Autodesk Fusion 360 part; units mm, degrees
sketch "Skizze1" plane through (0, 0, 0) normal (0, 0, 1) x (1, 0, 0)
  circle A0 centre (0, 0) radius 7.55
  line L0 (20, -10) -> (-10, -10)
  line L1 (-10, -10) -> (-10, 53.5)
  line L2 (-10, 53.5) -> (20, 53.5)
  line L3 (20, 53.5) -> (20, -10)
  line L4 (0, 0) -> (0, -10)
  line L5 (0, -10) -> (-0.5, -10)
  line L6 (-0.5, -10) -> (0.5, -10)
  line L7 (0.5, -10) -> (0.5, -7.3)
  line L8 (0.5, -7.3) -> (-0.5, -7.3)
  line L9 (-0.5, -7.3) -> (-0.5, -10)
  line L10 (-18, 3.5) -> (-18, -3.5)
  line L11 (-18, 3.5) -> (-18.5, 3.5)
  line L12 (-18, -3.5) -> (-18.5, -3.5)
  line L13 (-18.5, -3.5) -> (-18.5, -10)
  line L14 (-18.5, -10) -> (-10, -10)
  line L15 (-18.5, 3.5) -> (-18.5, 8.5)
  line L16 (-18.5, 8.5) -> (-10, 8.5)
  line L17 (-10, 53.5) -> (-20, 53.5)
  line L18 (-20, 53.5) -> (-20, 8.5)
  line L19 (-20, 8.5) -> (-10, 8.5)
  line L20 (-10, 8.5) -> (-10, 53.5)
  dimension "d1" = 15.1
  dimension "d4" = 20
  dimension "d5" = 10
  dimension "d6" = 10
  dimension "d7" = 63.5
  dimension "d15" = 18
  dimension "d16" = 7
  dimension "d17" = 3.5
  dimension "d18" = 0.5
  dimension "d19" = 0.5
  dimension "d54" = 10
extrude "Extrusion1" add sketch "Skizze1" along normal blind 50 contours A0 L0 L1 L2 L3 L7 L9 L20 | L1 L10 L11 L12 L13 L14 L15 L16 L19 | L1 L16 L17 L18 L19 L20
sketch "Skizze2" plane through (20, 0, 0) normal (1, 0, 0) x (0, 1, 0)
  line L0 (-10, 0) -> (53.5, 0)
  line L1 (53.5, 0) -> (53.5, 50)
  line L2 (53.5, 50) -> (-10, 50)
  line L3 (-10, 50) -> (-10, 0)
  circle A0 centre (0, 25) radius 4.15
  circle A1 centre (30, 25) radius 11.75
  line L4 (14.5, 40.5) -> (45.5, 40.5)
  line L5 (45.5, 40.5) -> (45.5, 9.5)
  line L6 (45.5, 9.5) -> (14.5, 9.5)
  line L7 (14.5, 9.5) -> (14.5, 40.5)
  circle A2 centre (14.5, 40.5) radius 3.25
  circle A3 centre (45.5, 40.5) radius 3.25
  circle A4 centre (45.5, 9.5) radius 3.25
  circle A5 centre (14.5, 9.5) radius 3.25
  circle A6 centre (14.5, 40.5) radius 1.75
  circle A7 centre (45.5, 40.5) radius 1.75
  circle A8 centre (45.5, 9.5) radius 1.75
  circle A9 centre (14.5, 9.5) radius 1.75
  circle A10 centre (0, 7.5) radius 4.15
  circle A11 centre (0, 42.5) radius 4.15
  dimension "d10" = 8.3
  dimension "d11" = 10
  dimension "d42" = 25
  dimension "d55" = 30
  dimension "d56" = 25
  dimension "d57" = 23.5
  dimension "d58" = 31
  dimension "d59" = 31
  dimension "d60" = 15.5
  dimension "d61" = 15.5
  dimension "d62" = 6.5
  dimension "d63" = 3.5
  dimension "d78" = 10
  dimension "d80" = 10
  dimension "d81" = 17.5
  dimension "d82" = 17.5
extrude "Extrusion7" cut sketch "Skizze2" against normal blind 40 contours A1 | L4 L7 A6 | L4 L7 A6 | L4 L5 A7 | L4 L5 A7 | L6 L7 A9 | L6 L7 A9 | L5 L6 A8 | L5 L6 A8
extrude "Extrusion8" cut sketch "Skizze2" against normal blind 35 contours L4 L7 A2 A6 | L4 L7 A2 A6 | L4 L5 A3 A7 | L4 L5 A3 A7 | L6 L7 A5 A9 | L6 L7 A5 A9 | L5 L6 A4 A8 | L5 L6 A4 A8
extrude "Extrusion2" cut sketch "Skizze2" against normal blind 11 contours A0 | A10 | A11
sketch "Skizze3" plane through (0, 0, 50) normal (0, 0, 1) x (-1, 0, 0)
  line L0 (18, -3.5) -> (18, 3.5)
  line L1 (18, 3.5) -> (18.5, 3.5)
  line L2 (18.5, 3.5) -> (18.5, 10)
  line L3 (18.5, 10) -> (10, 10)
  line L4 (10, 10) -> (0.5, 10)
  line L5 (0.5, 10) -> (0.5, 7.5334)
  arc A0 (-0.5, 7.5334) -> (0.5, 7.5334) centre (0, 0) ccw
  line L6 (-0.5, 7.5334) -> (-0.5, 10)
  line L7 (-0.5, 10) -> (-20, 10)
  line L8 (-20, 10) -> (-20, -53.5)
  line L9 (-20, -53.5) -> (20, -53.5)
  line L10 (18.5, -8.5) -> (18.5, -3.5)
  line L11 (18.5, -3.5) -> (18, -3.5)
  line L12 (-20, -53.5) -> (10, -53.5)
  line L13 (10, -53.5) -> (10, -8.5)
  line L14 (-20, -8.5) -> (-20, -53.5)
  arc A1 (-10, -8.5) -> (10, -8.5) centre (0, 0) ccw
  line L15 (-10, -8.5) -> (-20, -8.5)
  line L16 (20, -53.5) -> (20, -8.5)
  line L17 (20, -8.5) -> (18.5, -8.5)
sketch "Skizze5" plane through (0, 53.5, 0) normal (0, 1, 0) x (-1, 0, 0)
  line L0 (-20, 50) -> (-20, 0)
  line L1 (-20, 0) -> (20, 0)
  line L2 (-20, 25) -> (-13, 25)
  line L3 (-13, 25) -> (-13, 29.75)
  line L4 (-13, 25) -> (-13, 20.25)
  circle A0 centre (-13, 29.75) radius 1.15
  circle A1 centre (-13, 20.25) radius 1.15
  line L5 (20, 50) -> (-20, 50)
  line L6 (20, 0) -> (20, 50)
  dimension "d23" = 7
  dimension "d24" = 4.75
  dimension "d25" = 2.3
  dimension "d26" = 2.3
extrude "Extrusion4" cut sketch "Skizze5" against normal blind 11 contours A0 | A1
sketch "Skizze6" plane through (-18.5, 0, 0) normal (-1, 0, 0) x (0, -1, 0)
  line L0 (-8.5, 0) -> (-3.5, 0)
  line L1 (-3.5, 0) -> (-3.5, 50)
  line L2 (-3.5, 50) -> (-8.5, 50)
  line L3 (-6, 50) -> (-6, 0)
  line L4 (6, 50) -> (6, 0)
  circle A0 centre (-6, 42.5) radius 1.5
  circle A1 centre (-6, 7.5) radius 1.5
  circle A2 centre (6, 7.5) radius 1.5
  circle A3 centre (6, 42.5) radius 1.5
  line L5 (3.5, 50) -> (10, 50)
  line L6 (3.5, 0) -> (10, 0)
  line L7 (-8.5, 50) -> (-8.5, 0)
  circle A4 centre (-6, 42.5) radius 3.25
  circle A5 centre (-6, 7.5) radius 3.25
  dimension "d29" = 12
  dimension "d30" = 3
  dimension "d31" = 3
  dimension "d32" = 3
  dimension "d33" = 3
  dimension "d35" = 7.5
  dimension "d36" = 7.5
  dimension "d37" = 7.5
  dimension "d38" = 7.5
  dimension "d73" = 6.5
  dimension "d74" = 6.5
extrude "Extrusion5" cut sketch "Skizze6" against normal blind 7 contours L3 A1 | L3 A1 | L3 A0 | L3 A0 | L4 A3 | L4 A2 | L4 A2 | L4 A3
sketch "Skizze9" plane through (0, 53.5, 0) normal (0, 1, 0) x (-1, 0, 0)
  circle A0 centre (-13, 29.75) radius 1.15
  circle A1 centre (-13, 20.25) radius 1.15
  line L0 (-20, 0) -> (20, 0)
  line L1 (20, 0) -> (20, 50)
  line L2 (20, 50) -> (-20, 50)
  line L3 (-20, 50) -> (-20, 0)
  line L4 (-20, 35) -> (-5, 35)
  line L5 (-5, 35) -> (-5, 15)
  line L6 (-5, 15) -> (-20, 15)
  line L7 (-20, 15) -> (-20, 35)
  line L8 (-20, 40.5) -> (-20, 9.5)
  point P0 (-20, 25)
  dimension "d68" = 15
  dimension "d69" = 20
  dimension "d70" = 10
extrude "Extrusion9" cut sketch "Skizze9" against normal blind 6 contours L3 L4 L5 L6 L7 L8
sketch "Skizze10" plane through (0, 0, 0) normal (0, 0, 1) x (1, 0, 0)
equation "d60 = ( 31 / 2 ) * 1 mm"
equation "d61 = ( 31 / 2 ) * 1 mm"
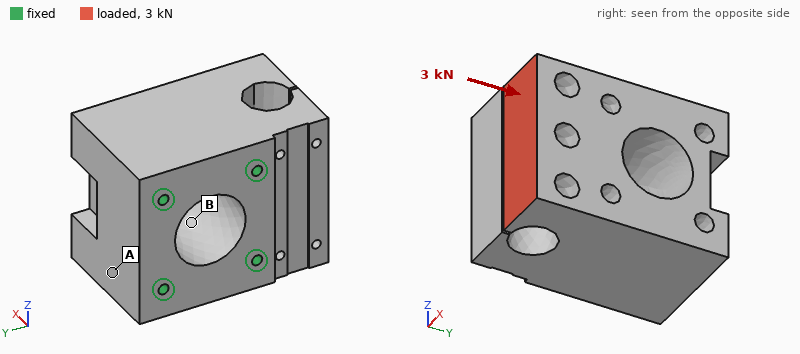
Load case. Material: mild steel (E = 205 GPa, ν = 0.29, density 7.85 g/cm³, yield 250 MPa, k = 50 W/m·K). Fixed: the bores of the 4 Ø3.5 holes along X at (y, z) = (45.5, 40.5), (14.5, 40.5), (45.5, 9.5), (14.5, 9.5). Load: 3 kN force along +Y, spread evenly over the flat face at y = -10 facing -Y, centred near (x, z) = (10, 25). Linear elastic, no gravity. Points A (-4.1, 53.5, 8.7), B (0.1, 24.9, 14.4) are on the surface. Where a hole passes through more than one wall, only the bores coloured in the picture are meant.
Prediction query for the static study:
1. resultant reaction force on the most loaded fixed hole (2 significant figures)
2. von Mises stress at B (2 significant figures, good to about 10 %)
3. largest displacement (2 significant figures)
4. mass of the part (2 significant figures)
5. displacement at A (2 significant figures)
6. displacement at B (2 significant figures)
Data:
1.5 kN
9.2 MPa
5.5 µm
710 g
2.1 µm
2.0 µm
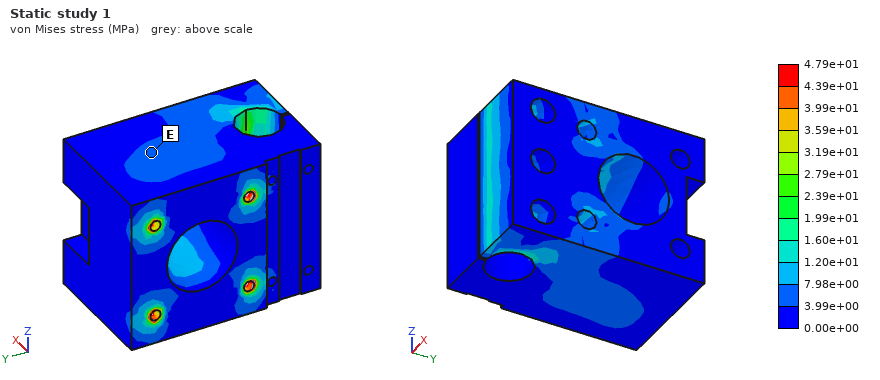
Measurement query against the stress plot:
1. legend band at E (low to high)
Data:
3.99e+00 to 7.98e+00 MPa
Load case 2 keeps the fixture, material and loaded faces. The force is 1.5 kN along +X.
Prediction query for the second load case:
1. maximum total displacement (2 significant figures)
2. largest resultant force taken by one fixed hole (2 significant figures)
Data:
8.7 µm
1.3 kN
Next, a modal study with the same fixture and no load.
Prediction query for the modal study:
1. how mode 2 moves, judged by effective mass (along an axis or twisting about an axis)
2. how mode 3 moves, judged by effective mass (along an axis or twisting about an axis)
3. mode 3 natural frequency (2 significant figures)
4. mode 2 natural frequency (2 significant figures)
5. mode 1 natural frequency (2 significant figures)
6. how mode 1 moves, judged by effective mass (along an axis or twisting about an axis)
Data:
along Z
twisting about X
12 kHz
7100 Hz
6400 Hz
along Y
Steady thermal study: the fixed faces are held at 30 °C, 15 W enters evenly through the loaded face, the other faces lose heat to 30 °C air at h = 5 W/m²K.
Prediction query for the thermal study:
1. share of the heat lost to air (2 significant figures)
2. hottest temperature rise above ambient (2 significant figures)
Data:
5.2 %
24 K
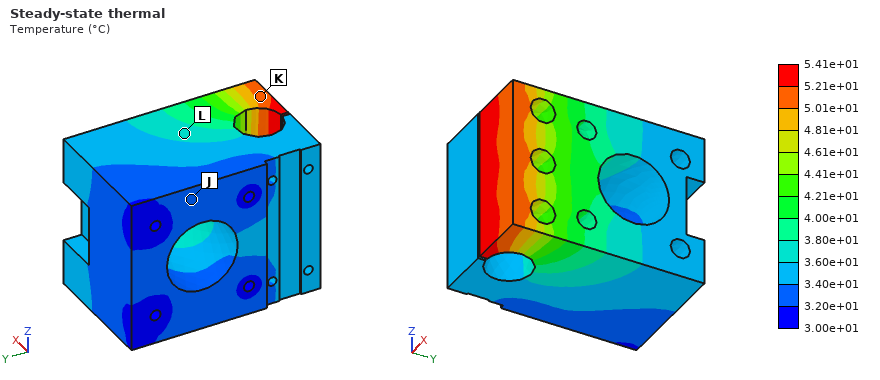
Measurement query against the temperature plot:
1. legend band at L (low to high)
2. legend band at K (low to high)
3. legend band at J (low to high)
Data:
3.60e+01 to 3.80e+01 °C
5.01e+01 to 5.21e+01 °C
3.20e+01 to 3.40e+01 °C
